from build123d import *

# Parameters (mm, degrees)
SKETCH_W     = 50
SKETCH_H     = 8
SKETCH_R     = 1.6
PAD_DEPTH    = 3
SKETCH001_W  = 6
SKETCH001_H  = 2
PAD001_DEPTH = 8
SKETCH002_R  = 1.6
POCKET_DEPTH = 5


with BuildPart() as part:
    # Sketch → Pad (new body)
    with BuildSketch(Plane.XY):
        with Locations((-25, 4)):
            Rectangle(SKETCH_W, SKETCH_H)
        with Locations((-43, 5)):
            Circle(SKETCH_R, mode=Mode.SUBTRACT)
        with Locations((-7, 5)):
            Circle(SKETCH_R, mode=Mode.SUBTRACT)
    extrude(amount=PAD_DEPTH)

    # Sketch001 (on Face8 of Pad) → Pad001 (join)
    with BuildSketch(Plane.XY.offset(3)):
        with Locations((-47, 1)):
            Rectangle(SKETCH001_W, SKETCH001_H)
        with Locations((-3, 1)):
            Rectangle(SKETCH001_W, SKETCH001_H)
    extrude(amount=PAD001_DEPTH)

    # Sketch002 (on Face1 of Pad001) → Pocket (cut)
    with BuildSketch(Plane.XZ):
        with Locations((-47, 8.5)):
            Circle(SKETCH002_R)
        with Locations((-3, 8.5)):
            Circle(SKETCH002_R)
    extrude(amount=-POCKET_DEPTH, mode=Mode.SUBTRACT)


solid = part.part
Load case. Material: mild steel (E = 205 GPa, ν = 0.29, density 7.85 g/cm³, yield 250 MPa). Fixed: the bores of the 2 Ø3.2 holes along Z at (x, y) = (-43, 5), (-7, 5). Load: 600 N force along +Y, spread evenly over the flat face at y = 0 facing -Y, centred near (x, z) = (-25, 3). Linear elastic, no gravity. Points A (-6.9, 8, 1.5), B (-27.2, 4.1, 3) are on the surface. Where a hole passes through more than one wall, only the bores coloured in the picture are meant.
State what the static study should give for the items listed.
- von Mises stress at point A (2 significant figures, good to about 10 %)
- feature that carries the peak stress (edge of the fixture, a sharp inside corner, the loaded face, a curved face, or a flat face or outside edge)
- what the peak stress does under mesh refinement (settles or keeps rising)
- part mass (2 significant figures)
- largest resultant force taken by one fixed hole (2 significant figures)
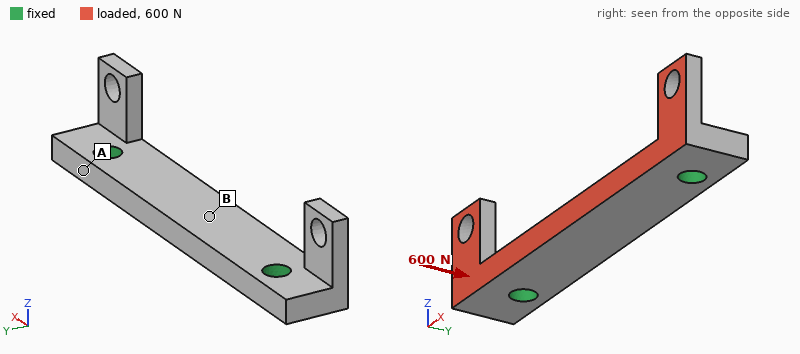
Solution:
18 MPa
a sharp inside corner
keeps rising
10 g
300 N
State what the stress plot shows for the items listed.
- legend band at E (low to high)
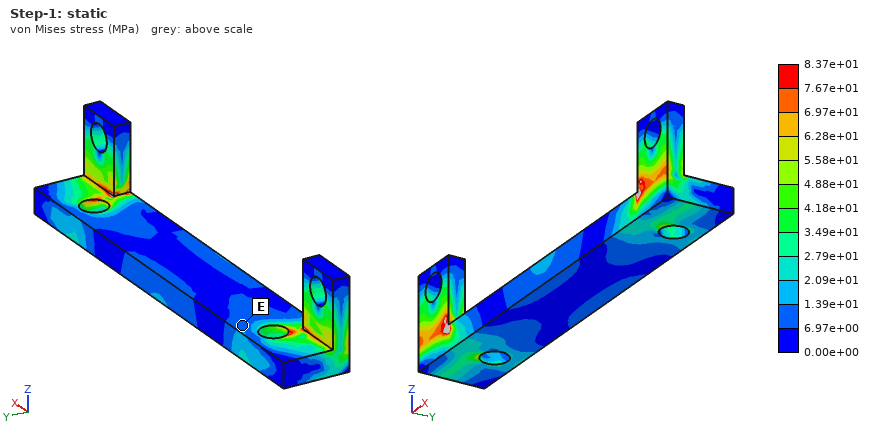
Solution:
6.97e+00 to 1.39e+01 MPa
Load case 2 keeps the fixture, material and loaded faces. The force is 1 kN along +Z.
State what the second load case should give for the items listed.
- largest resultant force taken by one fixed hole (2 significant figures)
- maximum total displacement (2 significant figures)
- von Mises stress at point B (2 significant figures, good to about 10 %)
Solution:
500 N
22 µm
51 MPa
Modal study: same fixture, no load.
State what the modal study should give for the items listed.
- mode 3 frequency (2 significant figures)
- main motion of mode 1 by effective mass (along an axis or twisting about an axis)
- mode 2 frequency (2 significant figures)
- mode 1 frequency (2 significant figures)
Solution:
19 kHz
along Z
19 kHz
13 kHz
